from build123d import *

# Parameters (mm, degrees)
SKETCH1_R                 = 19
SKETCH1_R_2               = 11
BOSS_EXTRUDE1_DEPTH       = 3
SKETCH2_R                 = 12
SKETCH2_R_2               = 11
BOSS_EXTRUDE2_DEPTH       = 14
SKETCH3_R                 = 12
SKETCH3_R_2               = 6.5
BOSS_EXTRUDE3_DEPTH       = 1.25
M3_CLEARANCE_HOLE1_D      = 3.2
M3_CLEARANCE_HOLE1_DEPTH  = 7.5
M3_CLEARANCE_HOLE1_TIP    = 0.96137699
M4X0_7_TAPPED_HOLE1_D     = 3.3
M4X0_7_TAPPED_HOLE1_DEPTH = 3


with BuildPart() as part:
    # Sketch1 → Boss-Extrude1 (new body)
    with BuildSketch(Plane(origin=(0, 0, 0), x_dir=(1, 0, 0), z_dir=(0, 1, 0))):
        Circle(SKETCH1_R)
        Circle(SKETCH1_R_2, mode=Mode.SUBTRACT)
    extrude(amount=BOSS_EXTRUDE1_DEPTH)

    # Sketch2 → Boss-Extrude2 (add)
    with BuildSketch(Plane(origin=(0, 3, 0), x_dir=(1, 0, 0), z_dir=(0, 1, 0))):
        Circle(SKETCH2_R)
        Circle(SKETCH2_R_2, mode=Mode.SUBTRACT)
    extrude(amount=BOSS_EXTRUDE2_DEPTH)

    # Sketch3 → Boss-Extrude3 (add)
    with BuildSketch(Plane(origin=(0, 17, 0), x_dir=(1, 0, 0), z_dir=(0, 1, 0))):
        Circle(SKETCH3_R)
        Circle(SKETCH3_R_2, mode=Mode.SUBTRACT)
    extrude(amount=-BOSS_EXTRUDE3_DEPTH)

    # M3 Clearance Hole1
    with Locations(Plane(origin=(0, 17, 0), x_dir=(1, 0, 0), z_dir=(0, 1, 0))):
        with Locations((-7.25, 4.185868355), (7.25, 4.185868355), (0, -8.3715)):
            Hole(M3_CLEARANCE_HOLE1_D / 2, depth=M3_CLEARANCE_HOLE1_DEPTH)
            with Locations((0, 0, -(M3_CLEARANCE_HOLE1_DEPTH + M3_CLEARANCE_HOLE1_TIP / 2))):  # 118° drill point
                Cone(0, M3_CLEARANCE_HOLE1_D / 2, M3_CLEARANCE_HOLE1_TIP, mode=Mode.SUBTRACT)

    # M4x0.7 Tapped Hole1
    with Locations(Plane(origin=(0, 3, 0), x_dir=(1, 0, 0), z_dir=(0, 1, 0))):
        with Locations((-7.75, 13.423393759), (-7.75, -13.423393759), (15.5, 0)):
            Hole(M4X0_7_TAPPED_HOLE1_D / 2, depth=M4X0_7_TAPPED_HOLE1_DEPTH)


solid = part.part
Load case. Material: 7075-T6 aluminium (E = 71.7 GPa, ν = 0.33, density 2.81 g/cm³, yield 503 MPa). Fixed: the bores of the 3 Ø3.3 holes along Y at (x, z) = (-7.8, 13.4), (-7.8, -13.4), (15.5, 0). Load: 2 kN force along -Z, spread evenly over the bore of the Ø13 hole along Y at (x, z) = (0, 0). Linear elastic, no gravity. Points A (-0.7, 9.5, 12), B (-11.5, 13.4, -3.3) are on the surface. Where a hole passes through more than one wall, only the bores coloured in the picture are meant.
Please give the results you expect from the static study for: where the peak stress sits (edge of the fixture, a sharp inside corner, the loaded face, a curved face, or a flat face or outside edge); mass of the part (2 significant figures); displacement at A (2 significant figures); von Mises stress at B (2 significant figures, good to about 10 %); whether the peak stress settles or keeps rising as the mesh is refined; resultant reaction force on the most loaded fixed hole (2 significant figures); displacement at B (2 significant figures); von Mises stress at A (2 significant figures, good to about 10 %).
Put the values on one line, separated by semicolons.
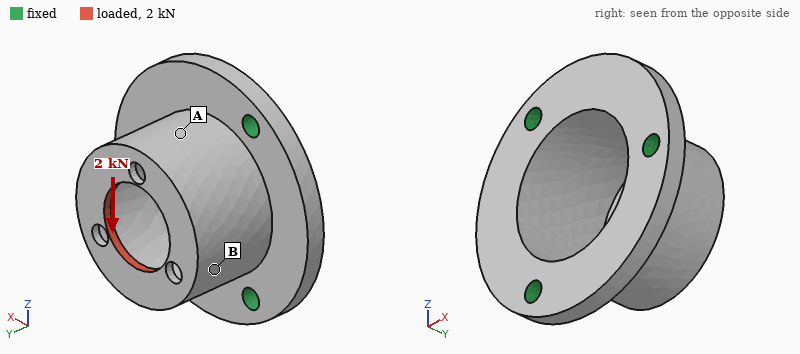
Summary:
a sharp inside corner; 9.8 g; 0.041 mm; 110 MPa; keeps rising; 1.4 kN; 0.046 mm; 41 MPa
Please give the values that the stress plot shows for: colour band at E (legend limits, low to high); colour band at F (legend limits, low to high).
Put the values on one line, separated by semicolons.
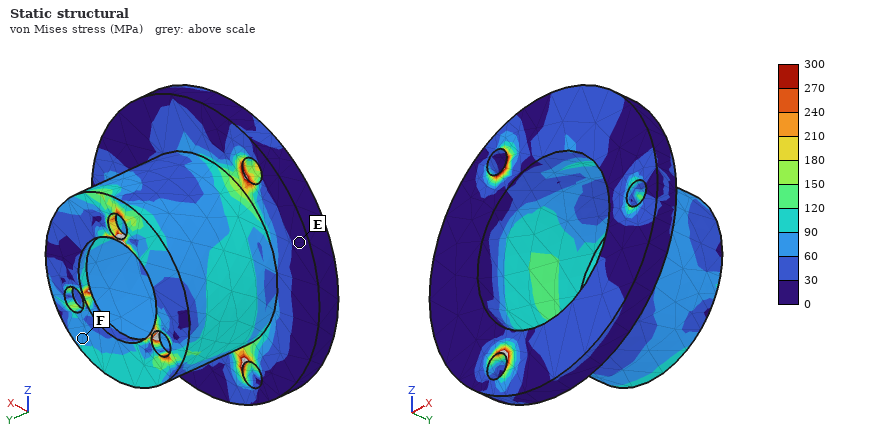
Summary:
0 to 30 MPa; 60 to 90 MPa
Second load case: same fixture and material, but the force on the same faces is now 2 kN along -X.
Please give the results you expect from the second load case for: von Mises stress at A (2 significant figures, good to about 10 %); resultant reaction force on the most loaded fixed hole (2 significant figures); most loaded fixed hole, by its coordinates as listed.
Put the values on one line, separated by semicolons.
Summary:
94 MPa; 1.5 kN; (15.5, 0)
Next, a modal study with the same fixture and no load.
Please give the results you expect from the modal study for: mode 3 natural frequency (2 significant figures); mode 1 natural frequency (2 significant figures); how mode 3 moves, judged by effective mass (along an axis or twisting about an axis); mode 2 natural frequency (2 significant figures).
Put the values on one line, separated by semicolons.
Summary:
19 kHz; 15 kHz; along Y; 15 kHz
